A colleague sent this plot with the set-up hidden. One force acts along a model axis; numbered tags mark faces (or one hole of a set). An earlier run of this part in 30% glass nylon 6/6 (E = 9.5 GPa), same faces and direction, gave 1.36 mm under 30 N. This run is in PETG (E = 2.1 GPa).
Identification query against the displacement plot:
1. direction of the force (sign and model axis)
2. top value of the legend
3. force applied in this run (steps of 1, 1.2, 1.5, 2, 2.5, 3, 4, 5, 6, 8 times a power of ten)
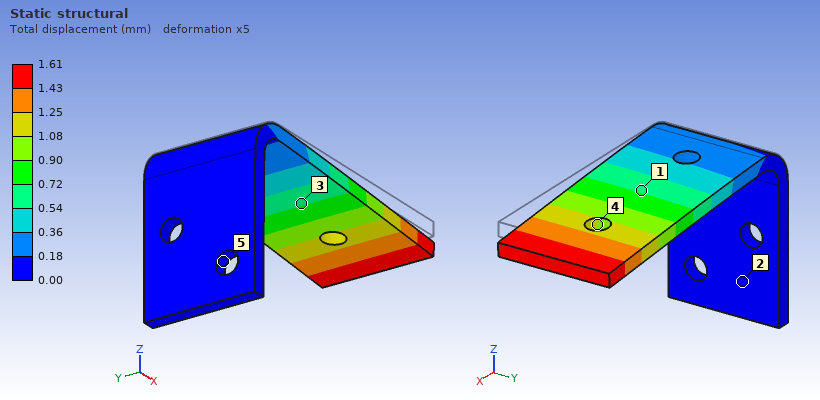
-Z
1.61 mm
8 N
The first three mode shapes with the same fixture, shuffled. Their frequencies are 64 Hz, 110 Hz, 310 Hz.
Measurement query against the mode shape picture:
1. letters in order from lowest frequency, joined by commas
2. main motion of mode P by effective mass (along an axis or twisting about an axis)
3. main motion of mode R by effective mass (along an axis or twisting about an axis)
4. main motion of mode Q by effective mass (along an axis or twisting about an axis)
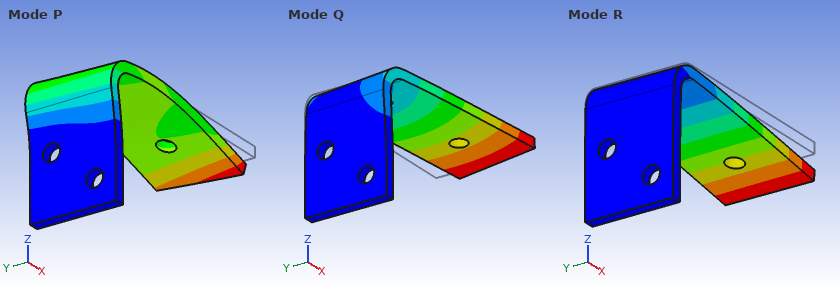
R, Q, P
along X
along Z
along Y
